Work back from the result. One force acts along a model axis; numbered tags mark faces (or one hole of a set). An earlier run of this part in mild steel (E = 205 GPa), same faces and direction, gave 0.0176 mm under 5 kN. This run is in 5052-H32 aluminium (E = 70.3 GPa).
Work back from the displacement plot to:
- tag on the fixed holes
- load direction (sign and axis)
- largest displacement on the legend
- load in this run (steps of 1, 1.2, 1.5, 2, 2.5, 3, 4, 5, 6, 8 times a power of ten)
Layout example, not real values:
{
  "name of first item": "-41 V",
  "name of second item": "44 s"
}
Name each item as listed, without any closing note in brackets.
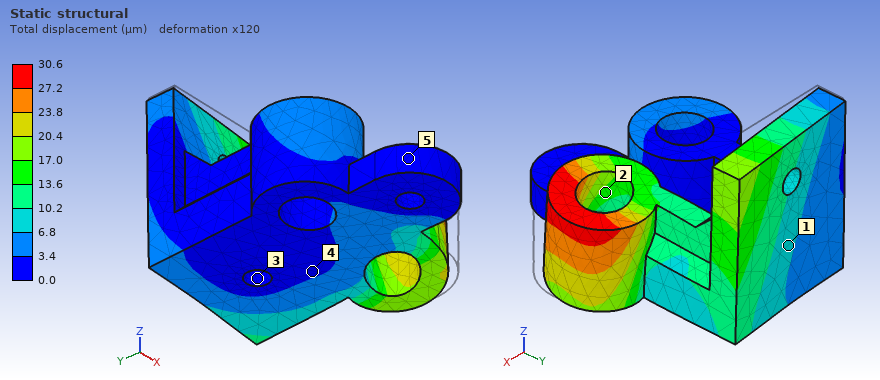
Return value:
{
  "tag on the fixed holes": "3",
  "load direction": "+Y",
  "largest displacement on the legend": "30.6 µm",
  "load in this run": "3 kN"
}
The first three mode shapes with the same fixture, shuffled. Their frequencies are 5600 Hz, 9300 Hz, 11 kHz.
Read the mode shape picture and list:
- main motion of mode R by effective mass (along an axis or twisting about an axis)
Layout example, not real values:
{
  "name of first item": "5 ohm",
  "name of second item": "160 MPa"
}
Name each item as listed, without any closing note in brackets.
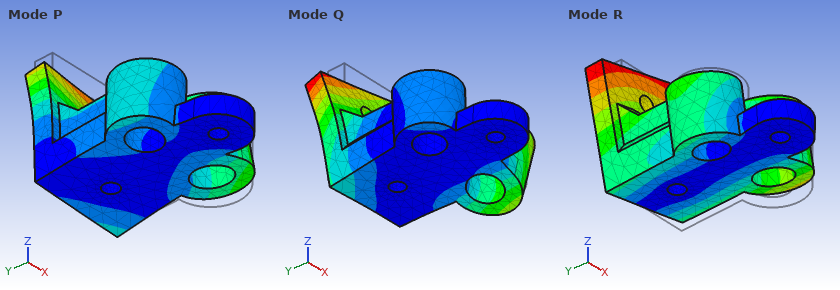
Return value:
{
  "main motion of mode R by effective mass": "along X"
}
